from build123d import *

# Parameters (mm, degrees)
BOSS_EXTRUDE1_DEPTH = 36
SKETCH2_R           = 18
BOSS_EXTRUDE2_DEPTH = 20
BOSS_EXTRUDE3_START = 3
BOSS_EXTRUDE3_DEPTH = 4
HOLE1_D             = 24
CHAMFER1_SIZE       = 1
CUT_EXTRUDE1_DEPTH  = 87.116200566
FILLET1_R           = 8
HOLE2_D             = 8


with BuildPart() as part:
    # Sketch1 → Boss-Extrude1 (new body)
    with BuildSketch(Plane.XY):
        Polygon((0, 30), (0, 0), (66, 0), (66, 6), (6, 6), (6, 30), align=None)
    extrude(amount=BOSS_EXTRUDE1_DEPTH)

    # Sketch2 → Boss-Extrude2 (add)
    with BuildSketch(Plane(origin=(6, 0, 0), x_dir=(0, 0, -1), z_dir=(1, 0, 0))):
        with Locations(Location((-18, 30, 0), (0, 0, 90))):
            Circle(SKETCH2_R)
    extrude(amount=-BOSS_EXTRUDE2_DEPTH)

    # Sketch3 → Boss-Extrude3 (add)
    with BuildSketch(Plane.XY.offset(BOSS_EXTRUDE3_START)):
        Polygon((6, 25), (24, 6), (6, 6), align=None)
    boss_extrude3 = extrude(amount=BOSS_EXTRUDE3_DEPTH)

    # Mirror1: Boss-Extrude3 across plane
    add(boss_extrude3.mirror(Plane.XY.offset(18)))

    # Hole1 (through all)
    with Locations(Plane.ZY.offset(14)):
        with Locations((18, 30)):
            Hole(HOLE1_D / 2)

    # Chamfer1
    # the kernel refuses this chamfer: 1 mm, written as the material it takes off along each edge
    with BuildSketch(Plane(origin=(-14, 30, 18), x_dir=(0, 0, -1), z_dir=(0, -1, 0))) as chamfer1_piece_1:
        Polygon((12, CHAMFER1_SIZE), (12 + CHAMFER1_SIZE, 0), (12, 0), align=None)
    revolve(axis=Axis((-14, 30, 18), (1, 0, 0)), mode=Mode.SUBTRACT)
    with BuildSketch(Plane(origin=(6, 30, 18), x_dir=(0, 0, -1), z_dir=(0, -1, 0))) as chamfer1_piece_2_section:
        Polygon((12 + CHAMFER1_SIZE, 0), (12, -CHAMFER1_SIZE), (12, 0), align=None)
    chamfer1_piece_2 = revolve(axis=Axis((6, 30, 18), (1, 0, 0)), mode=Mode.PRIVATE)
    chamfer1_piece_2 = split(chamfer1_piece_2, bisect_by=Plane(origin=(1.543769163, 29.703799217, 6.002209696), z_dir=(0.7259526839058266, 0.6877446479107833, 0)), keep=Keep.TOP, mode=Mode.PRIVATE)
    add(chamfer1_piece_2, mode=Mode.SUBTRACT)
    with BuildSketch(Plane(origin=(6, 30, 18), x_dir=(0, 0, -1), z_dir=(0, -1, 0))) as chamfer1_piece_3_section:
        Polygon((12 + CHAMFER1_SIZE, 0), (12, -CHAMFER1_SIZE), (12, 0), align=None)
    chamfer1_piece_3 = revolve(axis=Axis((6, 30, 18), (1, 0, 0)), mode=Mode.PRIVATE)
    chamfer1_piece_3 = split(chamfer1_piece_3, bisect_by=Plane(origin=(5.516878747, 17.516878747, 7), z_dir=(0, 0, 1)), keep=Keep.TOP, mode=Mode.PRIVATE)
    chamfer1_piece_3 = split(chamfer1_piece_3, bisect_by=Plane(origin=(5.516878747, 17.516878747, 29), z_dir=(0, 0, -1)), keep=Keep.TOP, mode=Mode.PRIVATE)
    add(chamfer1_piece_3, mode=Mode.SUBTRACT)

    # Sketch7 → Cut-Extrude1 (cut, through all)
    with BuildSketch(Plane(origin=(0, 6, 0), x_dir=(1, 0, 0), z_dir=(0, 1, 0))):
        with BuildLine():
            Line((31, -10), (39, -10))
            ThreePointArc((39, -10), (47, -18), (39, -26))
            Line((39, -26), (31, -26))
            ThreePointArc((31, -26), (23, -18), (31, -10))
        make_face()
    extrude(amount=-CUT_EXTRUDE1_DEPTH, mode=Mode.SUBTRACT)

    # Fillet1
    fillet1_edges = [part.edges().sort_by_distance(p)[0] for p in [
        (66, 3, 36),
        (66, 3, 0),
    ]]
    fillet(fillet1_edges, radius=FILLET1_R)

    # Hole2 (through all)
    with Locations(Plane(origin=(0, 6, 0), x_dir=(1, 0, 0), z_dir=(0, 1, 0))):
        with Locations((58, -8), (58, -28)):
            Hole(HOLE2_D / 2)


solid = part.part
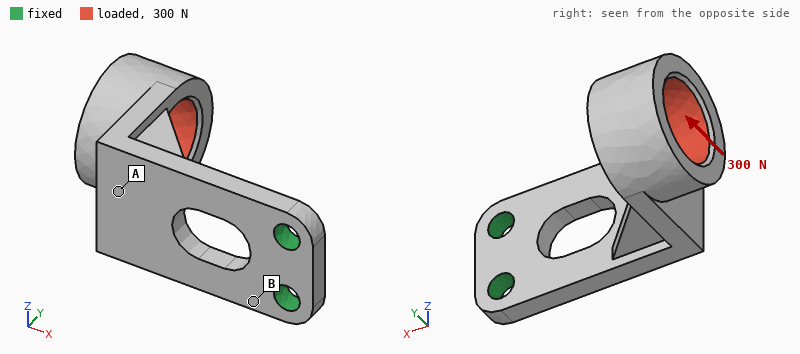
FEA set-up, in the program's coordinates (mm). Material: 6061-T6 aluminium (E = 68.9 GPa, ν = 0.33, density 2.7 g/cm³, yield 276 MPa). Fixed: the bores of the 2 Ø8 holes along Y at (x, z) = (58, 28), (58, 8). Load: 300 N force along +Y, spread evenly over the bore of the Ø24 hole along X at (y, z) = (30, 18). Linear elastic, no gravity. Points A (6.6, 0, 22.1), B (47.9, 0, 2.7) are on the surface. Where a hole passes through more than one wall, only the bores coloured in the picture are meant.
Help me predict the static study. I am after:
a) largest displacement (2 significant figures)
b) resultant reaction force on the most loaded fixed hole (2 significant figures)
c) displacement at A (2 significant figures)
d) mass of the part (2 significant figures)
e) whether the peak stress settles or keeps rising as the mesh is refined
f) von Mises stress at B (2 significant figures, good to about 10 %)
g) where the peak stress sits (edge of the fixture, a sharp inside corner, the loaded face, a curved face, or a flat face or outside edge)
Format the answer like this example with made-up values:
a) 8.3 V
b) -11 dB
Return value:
a) 1.1 mm
b) 150 N
c) 0.49 mm
d) 71 g
e) keeps rising
f) 93 MPa
g) edge of the fixture
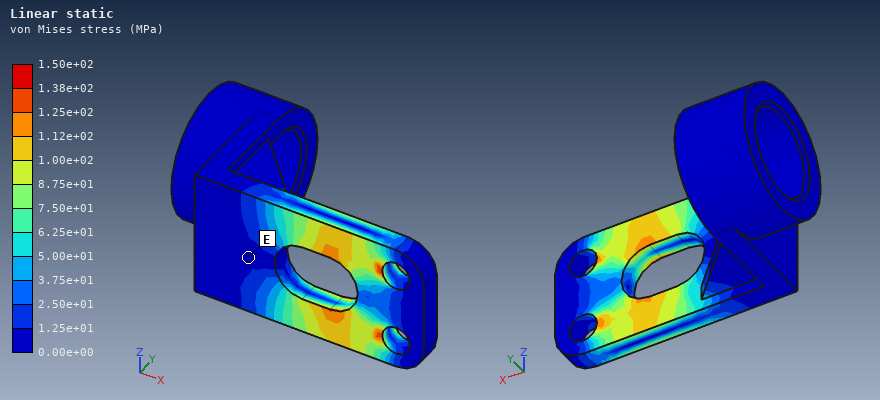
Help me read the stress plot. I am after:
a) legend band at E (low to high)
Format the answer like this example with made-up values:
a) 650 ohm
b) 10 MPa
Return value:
a) 0.00e+00 to 1.25e+01 MPa
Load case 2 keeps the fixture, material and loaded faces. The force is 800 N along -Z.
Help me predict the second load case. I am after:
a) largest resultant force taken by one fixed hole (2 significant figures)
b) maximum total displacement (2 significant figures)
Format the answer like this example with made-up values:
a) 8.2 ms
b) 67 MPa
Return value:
a) 2.0 kN
b) 0.70 mm
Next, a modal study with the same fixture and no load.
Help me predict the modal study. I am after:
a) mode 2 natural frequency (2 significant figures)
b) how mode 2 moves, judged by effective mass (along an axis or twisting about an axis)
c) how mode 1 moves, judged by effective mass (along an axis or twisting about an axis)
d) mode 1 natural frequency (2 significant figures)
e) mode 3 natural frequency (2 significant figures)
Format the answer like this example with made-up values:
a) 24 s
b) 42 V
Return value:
a) 1000 Hz
b) along Z
c) along Y
d) 450 Hz
e) 2800 Hz
